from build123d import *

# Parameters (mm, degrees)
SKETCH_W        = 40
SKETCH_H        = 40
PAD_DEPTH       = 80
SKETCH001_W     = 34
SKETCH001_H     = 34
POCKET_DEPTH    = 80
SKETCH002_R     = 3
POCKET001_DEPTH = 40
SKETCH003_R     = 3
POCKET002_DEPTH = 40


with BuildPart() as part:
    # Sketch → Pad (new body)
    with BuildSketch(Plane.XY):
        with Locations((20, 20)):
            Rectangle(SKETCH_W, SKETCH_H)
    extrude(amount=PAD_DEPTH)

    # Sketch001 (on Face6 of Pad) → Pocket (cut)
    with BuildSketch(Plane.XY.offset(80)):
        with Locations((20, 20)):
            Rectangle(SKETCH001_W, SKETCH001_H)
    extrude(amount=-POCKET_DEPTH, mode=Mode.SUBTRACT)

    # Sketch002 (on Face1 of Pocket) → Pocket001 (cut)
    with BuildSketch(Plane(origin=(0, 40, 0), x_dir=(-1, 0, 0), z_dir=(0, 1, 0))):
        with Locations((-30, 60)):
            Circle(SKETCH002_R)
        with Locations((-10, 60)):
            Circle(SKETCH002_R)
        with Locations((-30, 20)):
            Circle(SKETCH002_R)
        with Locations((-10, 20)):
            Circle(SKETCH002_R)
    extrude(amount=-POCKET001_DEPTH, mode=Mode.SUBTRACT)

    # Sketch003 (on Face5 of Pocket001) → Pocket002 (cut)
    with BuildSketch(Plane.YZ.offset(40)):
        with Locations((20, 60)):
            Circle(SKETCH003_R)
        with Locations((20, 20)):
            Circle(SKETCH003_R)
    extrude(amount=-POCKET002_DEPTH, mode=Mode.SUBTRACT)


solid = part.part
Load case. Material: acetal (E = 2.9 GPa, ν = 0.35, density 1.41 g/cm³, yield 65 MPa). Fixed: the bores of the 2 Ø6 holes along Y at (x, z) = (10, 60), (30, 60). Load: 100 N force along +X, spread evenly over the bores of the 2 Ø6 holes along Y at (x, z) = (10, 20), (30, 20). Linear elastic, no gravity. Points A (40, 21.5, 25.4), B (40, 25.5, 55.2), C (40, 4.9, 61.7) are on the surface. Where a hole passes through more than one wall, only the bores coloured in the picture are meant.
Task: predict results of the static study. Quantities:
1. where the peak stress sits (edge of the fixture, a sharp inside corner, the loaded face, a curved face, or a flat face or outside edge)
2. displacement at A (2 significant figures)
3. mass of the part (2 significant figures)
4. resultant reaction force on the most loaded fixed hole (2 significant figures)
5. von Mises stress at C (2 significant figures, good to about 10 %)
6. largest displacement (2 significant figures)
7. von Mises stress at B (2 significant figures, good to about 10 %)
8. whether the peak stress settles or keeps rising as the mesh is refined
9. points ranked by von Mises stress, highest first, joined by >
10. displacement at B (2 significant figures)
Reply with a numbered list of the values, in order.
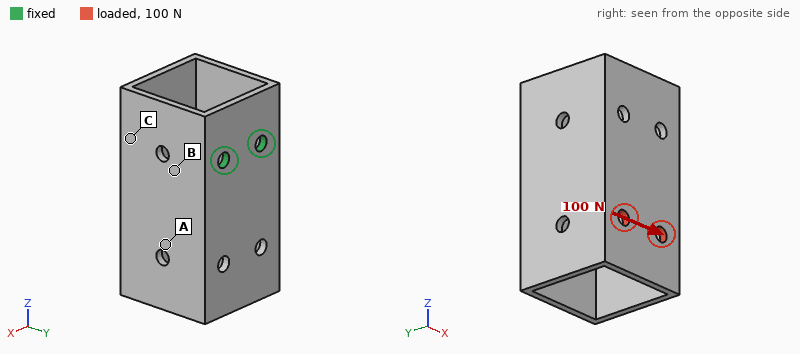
1. edge of the fixture
2. 0.53 mm
3. 49 g
4. 200 N
5. 5.0 MPa
6. 1.1 mm
7. 3.2 MPa
8. keeps rising
9. C > B > A
10. 0.39 mm
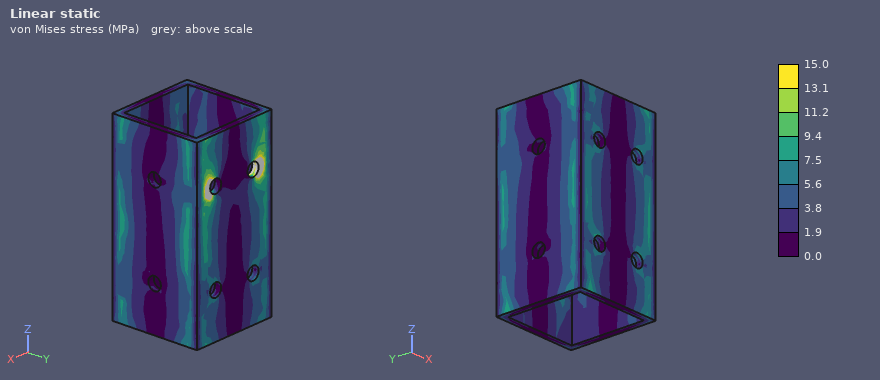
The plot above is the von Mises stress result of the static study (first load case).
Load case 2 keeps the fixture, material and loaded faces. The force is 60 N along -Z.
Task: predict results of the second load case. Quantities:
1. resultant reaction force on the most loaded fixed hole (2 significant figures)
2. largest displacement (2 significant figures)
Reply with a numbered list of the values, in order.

1. 30 N
2. 1.2 mm
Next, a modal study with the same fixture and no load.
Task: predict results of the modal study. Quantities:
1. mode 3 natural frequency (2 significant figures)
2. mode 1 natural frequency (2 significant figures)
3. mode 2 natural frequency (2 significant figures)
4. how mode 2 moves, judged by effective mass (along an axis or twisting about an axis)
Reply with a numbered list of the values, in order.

1. 670 Hz
2. 220 Hz
3. 320 Hz
4. along X
